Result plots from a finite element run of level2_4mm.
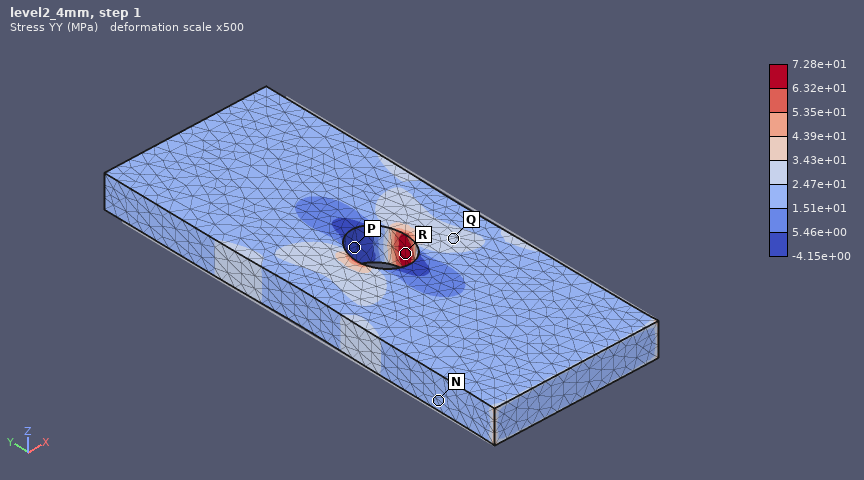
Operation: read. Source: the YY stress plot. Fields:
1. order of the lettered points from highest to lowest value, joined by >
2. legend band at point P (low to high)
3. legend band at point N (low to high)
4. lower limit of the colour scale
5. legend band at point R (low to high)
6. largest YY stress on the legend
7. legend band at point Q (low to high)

R > Q > N > P
-4.15e+00 to 5.46e+00 MPa
1.51e+01 to 2.47e+01 MPa
-4.15e+00 MPa
6.32e+01 to 7.28e+01 MPa
7.28e+01 MPa
2.47e+01 to 3.43e+01 MPa
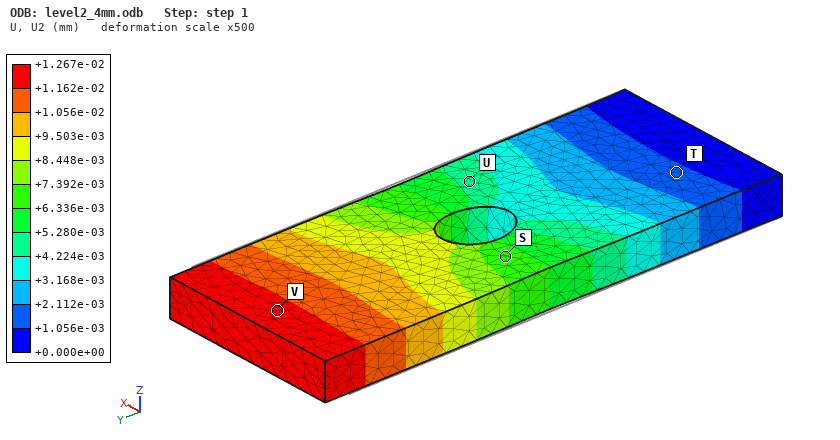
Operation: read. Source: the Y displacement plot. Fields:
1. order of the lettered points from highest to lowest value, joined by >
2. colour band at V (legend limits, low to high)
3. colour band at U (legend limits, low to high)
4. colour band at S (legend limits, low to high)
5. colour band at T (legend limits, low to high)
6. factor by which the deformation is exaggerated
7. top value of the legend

V > S > U > T
+1.162e-02 to +1.267e-02 mm
+4.224e-03 to +5.280e-03 mm
+6.336e-03 to +7.392e-03 mm
+1.056e-03 to +2.112e-03 mm
500
+1.267e-02 mm
